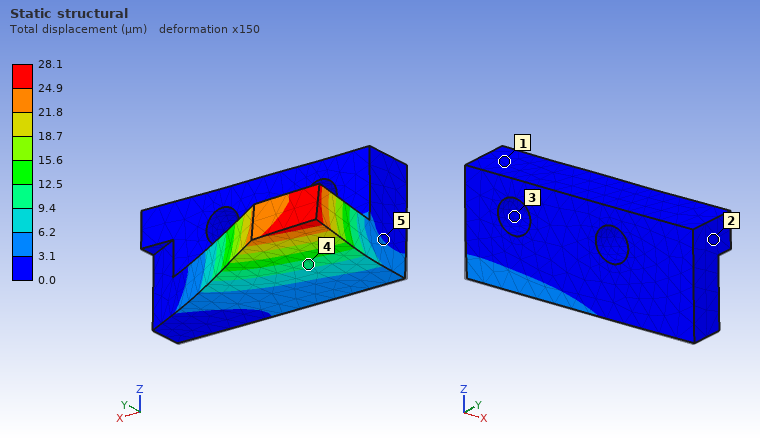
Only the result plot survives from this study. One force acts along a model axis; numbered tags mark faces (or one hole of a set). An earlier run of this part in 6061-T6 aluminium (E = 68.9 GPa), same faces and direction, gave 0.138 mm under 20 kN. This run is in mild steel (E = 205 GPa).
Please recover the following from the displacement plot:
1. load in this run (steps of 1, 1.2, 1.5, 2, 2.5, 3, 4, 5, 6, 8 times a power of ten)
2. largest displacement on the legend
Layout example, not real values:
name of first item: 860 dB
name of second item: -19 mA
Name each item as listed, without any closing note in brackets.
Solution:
load in this run: 12 kN
largest displacement on the legend: 28.1 µm
